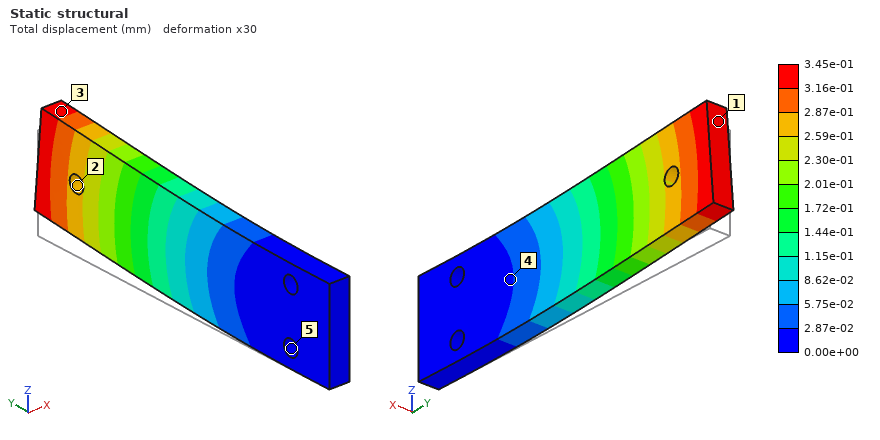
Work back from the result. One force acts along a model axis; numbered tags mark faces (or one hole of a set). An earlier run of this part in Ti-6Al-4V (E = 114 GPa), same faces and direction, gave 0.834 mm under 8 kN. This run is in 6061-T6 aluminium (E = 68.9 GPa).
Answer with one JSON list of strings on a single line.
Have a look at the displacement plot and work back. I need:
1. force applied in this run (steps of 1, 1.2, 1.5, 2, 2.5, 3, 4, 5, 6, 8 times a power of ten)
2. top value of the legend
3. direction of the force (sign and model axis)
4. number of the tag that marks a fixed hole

["2 kN", "3.45e-01 mm", "+Z", "5"]
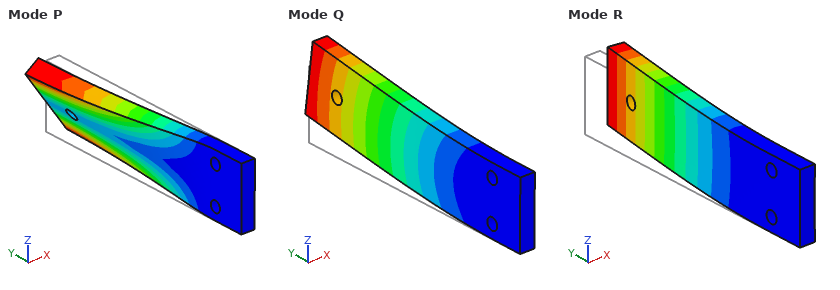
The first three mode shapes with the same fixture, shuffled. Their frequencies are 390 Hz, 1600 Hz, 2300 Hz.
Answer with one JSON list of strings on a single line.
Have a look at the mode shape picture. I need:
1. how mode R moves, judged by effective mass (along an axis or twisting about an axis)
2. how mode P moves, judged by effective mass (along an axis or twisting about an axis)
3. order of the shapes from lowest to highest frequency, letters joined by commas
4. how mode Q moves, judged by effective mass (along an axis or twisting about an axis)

["along X", "twisting about Y", "R, Q, P", "along Z"]
